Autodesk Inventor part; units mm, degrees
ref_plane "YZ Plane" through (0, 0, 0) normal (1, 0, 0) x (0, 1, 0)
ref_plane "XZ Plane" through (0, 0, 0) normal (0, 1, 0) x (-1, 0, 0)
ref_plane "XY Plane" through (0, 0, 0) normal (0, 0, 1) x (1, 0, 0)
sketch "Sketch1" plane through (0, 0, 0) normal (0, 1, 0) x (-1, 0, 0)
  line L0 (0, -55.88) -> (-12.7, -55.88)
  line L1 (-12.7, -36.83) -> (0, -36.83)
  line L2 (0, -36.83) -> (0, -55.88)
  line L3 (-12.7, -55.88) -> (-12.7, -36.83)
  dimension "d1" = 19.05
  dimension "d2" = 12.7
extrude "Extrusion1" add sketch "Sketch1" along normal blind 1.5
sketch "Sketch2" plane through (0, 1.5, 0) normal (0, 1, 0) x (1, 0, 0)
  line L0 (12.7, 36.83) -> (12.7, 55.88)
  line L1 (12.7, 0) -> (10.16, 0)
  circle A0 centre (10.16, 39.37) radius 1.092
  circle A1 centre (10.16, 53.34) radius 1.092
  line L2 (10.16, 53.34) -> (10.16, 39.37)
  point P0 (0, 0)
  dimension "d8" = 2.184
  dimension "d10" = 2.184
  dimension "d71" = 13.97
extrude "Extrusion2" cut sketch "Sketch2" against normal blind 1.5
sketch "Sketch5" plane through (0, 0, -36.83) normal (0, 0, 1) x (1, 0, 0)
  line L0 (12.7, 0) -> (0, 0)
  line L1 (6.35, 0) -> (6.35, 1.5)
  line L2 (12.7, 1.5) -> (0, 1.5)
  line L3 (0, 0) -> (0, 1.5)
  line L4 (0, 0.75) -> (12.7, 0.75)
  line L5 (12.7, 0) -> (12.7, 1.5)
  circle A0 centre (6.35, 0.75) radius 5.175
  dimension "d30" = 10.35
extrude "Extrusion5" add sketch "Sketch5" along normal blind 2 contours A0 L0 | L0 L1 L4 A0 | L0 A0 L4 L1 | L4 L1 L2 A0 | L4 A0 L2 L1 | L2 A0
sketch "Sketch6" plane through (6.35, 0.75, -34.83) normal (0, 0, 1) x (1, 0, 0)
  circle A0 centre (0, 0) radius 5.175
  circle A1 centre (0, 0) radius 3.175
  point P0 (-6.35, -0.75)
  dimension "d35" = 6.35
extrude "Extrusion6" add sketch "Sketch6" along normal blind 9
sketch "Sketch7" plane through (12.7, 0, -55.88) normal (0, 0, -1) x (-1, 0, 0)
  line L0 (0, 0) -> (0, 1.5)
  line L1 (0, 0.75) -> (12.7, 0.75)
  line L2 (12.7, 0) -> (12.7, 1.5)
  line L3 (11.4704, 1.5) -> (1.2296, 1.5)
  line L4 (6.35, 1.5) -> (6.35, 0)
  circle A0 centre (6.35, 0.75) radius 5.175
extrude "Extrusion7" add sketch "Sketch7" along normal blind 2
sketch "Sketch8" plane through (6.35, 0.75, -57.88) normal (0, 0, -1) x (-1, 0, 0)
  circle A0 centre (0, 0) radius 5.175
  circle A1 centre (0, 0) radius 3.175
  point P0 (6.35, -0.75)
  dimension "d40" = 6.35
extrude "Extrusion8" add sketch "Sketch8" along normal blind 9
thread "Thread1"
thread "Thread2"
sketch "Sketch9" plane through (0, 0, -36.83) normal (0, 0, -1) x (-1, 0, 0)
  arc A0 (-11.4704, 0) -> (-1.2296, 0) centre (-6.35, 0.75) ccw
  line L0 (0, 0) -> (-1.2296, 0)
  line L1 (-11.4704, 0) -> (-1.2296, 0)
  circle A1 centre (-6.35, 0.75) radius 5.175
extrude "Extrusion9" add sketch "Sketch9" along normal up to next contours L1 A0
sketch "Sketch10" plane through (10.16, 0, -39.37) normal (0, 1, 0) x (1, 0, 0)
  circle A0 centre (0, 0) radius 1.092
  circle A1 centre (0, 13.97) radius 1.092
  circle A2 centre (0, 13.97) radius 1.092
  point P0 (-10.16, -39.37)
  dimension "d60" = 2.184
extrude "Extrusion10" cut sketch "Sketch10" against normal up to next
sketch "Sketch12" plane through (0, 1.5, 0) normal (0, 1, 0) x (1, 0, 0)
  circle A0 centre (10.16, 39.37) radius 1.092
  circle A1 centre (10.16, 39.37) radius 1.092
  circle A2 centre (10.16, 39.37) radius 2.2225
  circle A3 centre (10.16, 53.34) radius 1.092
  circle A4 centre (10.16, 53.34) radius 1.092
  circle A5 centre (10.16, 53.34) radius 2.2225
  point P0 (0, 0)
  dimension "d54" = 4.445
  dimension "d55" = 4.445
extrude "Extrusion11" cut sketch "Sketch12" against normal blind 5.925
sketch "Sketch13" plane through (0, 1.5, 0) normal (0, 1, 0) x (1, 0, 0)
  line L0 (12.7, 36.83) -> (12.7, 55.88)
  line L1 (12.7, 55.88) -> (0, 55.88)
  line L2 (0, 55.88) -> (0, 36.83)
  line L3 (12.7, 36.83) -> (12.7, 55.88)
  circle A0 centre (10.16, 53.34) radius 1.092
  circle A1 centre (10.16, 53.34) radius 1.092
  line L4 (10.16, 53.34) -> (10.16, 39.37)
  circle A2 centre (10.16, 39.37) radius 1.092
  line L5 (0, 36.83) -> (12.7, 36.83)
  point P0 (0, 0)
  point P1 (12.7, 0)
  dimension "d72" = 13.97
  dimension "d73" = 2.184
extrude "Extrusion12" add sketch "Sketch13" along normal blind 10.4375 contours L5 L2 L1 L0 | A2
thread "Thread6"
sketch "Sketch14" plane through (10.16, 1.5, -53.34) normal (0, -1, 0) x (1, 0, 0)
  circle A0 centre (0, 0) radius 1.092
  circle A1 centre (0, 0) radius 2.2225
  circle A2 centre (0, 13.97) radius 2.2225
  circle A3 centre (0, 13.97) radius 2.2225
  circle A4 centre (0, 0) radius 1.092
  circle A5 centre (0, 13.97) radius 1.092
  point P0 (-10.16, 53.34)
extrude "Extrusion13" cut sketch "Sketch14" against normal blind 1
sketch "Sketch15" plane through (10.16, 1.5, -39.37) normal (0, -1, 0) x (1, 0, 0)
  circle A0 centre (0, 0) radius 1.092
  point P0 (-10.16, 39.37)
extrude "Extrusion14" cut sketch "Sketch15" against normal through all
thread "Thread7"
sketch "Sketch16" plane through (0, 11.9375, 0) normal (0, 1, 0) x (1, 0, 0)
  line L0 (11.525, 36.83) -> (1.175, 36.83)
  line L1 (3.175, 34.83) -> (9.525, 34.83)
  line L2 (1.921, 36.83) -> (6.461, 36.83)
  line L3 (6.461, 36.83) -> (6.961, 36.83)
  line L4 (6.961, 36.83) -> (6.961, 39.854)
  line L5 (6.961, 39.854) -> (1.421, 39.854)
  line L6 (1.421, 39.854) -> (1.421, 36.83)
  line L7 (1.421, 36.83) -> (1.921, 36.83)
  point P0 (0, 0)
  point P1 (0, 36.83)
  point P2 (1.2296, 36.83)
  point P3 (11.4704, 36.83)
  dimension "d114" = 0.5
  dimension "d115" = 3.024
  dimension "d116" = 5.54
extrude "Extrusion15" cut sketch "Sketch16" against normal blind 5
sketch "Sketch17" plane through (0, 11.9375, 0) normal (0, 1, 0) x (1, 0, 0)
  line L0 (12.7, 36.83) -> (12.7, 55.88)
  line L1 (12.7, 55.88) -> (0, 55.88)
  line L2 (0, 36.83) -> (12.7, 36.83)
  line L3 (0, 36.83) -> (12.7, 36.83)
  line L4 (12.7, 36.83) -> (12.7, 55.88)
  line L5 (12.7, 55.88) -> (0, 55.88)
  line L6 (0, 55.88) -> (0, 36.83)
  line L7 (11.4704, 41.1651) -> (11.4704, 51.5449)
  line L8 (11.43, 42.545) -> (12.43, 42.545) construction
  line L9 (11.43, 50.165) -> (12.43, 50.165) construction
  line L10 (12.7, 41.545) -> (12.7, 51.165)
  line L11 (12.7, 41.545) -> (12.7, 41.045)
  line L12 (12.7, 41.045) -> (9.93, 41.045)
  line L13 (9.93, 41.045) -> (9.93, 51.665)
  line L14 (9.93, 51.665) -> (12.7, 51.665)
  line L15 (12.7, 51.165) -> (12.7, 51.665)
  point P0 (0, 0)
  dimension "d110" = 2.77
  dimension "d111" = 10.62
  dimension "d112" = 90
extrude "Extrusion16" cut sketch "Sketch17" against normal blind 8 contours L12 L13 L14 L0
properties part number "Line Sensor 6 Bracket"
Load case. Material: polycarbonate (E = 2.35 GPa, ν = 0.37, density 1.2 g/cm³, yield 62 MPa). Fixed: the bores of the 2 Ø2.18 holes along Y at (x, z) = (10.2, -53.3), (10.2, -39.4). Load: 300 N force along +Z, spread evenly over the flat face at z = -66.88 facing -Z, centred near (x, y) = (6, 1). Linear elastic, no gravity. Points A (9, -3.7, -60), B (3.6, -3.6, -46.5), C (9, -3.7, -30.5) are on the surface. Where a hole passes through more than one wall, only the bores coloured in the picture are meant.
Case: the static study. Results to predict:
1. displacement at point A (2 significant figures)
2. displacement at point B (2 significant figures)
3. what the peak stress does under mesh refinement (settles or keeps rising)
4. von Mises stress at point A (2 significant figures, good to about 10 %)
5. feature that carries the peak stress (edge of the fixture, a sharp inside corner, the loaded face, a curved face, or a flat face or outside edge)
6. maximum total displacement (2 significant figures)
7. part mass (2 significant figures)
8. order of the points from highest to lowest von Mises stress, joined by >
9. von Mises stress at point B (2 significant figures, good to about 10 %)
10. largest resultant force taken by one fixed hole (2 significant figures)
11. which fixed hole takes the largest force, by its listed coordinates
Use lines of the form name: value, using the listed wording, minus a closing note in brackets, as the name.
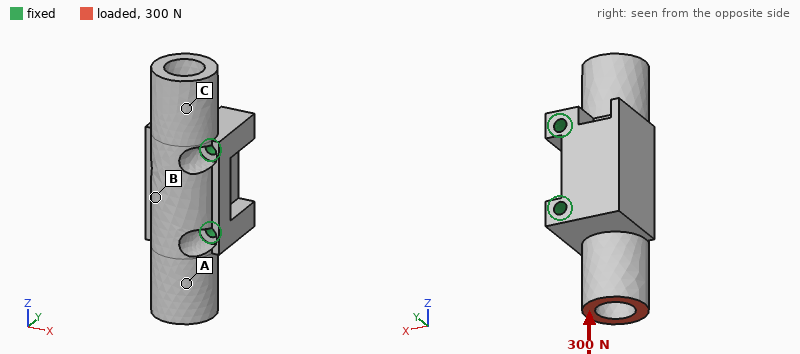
displacement at point A: 61 µm
displacement at point B: 23 µm
what the peak stress does under mesh refinement: keeps rising
von Mises stress at point A: 5.1 MPa
feature that carries the peak stress: edge of the fixture
maximum total displacement: 90 µm
part mass: 5.1 g
order of the points from highest to lowest von Mises stress, joined by >: A > B > C
von Mises stress at point B: 2.7 MPa
largest resultant force taken by one fixed hole: 220 N
which fixed hole takes the largest force, by its listed coordinates: (10.2, -53.3)
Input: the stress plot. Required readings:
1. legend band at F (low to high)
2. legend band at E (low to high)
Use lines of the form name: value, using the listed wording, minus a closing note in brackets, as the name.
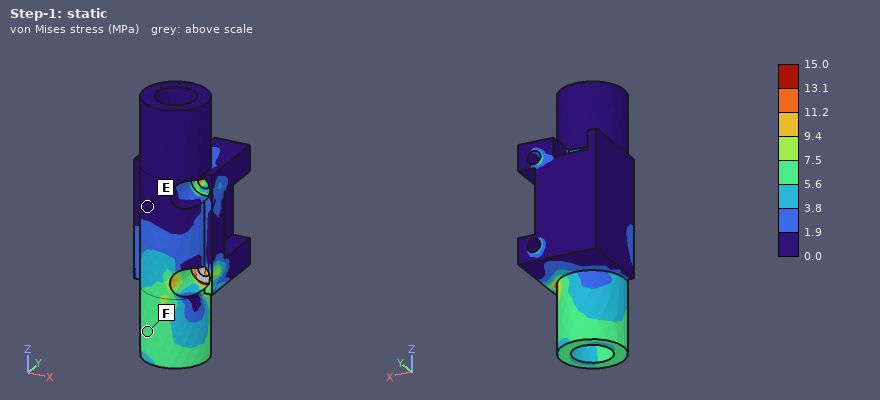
legend band at F: 5.6 to 7.5 MPa
legend band at E: 0.0 to 1.9 MPa
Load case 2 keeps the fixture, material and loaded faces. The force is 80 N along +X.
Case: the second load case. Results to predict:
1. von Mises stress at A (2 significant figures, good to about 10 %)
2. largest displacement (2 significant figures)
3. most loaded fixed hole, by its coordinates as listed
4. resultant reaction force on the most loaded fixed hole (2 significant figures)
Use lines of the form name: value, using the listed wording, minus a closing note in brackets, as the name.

von Mises stress at A: 3.3 MPa
largest displacement: 0.16 mm
most loaded fixed hole, by its coordinates as listed: (10.2, -53.3)
resultant reaction force on the most loaded fixed hole: 160 N
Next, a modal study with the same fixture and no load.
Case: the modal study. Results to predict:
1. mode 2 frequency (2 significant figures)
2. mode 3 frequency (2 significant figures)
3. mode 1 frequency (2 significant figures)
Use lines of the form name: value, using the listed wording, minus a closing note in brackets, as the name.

mode 2 frequency: 6000 Hz
mode 3 frequency: 6800 Hz
mode 1 frequency: 5800 Hz
